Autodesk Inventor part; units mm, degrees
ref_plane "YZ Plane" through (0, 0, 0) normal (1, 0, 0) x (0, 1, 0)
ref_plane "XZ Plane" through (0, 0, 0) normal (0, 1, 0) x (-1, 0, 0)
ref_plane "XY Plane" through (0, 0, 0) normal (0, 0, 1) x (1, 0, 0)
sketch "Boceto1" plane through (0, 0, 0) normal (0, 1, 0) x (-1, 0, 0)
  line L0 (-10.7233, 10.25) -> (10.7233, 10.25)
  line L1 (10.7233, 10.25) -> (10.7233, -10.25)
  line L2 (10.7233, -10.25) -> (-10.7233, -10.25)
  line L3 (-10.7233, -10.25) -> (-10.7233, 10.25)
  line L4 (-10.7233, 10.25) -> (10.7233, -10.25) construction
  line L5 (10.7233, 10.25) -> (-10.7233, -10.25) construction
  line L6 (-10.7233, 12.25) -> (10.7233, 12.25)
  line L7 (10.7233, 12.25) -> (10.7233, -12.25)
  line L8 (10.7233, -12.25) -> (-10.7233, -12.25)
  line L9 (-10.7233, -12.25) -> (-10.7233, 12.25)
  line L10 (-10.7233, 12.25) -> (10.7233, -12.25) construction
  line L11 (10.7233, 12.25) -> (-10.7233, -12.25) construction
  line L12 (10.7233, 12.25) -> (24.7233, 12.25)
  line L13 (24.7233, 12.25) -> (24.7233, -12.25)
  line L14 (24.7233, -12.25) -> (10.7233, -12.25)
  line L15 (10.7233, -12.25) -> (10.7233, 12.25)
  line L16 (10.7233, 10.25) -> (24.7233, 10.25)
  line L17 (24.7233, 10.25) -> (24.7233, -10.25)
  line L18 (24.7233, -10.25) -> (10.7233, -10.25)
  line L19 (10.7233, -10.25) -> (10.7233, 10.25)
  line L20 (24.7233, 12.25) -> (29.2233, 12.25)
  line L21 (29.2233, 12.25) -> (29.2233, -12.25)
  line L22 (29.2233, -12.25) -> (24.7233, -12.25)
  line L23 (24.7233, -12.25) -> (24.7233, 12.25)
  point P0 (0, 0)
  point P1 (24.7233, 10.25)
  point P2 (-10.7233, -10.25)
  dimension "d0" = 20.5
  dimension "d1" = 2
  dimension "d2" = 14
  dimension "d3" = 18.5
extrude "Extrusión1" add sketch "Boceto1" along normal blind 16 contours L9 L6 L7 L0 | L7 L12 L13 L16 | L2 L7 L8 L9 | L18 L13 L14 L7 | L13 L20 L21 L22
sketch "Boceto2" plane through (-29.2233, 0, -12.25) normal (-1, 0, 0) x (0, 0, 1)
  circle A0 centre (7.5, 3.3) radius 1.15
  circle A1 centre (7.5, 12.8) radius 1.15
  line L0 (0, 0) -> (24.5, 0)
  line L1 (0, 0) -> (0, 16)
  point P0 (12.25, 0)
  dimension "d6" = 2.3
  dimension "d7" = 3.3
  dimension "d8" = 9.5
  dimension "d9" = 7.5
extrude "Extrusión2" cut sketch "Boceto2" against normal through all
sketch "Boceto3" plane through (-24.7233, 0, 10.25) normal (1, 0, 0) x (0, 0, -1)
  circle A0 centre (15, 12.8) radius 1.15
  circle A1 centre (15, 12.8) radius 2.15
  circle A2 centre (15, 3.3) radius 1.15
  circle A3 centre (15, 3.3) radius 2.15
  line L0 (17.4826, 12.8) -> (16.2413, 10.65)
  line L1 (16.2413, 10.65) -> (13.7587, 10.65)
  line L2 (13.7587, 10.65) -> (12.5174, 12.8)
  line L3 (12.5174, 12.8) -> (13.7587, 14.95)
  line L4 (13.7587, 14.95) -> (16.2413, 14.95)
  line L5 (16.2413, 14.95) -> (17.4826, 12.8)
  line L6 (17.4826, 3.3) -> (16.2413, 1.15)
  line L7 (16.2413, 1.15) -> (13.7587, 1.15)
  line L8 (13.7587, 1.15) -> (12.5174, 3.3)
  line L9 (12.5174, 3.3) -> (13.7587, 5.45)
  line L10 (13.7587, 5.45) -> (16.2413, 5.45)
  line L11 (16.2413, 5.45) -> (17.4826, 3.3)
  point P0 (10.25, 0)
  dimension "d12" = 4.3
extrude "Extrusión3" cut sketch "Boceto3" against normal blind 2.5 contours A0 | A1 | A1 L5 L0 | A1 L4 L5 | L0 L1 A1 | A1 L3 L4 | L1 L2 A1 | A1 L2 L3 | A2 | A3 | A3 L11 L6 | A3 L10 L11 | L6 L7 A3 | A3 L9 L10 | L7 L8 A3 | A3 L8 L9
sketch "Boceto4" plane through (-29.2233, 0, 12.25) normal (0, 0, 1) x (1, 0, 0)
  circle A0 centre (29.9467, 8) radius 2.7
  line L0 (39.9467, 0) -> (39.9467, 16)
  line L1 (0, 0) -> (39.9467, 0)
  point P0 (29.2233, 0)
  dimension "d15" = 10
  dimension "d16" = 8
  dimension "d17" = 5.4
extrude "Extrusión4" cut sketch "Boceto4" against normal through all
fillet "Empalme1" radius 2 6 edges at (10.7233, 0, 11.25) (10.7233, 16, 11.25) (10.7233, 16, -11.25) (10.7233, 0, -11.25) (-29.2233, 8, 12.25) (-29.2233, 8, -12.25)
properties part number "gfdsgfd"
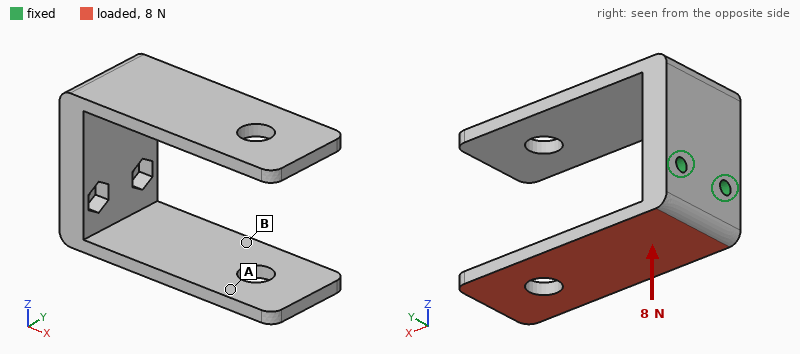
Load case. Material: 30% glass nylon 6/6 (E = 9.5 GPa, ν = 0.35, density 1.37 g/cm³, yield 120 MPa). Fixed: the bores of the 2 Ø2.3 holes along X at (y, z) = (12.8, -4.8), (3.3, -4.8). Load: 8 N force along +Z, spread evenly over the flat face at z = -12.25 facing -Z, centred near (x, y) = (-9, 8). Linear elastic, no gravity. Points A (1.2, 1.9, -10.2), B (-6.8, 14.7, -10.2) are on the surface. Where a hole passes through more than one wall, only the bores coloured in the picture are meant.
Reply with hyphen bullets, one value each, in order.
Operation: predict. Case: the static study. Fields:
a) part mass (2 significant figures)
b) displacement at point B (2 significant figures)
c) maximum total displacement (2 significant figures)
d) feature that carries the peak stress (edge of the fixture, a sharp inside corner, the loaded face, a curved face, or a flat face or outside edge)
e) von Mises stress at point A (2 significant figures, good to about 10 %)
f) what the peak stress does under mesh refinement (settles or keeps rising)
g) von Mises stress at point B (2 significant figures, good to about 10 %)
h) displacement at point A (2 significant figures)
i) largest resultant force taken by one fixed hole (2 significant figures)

- 5.2 g
- 0.20 mm
- 0.50 mm
- edge of the fixture
- 1.3 MPa
- keeps rising
- 3.0 MPa
- 0.33 mm
- 4.0 N
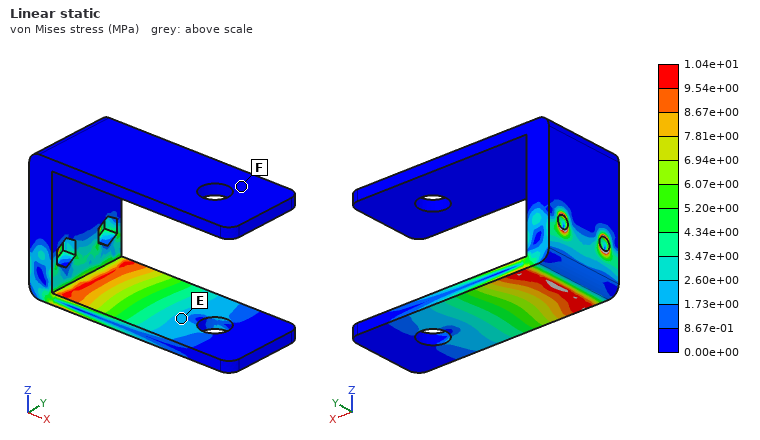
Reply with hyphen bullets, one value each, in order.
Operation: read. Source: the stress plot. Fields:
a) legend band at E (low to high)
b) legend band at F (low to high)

- 1.73e+00 to 2.60e+00 MPa
- 0.00e+00 to 8.67e-01 MPa
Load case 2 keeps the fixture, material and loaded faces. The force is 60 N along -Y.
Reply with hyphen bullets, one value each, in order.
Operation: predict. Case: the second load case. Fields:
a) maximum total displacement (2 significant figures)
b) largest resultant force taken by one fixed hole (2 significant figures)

- 0.23 mm
- 120 N
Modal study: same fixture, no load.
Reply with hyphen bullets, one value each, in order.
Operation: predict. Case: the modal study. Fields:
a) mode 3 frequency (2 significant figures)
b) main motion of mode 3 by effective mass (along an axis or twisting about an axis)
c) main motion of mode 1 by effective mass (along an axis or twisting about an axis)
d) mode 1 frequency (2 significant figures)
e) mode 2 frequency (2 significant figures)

- 1600 Hz
- along Y
- along Z
- 590 Hz
- 640 Hz
